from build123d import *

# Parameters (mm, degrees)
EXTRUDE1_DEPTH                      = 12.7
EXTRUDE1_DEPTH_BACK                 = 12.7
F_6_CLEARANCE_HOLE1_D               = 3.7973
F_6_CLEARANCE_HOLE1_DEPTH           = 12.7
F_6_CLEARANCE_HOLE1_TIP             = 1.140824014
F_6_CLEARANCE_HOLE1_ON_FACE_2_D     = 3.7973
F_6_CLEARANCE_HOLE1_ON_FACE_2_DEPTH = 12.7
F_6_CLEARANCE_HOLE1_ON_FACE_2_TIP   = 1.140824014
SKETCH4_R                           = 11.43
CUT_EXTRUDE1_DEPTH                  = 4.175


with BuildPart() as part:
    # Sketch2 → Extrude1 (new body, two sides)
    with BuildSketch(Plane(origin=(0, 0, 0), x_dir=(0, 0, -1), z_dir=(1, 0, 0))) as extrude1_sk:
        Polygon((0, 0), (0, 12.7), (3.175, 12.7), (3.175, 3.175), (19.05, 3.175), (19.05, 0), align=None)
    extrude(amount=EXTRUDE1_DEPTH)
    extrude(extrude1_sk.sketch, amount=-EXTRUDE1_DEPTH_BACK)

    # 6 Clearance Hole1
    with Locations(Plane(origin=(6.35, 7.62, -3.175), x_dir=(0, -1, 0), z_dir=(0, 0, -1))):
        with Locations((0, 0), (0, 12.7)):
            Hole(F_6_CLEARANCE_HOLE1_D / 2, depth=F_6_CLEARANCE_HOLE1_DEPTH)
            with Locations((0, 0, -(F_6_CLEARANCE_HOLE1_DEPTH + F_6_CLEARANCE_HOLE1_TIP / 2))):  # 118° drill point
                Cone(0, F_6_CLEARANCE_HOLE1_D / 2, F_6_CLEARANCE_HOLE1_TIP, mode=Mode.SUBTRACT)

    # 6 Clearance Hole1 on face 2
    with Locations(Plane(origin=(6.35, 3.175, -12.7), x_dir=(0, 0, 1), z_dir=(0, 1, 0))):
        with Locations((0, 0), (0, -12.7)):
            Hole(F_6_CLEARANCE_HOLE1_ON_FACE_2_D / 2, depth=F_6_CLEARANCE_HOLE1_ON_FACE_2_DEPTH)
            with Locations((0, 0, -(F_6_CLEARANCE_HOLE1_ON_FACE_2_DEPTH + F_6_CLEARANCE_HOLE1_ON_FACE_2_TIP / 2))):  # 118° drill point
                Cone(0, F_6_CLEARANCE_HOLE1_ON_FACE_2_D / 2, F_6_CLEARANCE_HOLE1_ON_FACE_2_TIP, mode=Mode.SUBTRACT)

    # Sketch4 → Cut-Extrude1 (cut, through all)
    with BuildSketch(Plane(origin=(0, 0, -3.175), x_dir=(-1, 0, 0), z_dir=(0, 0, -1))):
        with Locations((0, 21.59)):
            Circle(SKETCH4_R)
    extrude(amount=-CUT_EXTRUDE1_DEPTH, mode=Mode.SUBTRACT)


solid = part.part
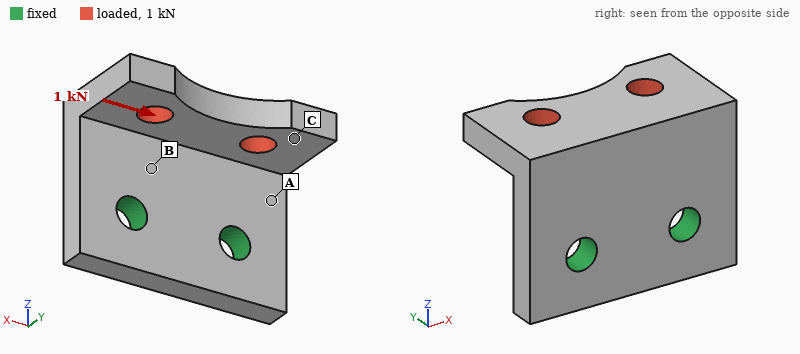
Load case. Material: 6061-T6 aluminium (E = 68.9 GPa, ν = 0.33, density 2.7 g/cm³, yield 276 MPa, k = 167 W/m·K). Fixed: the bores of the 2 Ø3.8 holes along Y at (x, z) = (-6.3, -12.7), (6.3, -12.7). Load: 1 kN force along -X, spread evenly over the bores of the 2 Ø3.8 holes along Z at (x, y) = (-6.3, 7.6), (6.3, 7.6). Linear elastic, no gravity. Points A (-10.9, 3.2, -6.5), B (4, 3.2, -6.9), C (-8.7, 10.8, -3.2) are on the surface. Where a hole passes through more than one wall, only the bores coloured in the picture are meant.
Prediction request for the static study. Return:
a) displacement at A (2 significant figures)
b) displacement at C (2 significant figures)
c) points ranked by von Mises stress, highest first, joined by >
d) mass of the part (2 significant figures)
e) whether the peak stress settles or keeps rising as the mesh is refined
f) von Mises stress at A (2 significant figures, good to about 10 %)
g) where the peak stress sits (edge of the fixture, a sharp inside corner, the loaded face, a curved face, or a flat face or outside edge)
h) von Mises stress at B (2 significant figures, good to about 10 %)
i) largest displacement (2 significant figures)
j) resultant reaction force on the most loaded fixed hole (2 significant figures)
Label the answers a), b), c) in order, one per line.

a) 21 µm
b) 56 µm
c) B > A > C
d) 5.6 g
e) keeps rising
f) 53 MPa
g) edge of the fixture
h) 86 MPa
i) 73 µm
j) 900 N
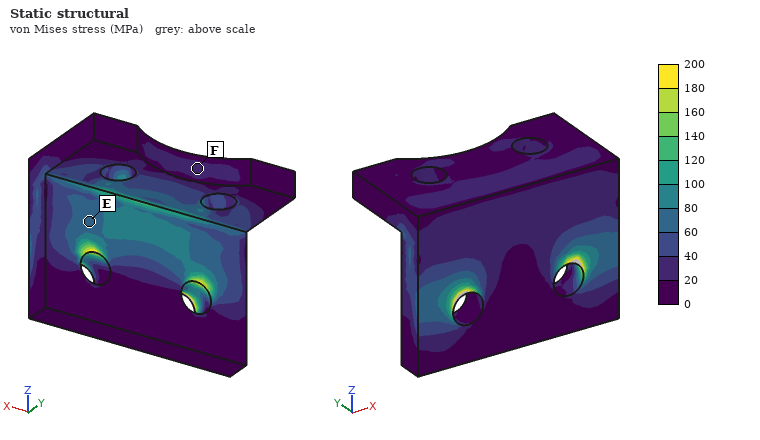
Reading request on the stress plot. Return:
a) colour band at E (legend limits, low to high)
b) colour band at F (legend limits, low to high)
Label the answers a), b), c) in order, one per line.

a) 60 to 80 MPa
b) 20 to 40 MPa
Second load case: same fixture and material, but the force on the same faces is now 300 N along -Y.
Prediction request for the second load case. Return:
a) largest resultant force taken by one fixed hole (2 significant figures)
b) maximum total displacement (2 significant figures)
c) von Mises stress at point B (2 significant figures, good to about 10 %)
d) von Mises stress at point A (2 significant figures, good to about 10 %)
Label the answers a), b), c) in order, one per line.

a) 150 N
b) 48 µm
c) 34 MPa
d) 32 MPa
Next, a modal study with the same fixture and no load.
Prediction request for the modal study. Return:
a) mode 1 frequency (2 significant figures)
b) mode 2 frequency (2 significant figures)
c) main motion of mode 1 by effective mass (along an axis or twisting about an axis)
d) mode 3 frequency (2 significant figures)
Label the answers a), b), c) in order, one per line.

a) 8500 Hz
b) 13 kHz
c) along Y
d) 22 kHz
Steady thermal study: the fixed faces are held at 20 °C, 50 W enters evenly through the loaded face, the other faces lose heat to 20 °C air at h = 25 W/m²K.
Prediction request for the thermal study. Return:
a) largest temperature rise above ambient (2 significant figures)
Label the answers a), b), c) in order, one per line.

a) 67 K
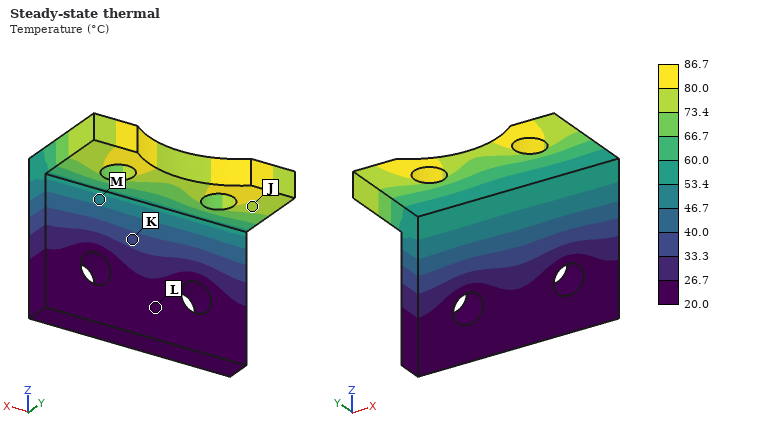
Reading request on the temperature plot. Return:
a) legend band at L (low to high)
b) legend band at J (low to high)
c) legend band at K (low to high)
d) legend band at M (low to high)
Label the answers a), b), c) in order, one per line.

a) 20.0 to 26.7 °C
b) 73.4 to 80.0 °C
c) 33.3 to 40.0 °C
d) 46.7 to 53.4 °C
